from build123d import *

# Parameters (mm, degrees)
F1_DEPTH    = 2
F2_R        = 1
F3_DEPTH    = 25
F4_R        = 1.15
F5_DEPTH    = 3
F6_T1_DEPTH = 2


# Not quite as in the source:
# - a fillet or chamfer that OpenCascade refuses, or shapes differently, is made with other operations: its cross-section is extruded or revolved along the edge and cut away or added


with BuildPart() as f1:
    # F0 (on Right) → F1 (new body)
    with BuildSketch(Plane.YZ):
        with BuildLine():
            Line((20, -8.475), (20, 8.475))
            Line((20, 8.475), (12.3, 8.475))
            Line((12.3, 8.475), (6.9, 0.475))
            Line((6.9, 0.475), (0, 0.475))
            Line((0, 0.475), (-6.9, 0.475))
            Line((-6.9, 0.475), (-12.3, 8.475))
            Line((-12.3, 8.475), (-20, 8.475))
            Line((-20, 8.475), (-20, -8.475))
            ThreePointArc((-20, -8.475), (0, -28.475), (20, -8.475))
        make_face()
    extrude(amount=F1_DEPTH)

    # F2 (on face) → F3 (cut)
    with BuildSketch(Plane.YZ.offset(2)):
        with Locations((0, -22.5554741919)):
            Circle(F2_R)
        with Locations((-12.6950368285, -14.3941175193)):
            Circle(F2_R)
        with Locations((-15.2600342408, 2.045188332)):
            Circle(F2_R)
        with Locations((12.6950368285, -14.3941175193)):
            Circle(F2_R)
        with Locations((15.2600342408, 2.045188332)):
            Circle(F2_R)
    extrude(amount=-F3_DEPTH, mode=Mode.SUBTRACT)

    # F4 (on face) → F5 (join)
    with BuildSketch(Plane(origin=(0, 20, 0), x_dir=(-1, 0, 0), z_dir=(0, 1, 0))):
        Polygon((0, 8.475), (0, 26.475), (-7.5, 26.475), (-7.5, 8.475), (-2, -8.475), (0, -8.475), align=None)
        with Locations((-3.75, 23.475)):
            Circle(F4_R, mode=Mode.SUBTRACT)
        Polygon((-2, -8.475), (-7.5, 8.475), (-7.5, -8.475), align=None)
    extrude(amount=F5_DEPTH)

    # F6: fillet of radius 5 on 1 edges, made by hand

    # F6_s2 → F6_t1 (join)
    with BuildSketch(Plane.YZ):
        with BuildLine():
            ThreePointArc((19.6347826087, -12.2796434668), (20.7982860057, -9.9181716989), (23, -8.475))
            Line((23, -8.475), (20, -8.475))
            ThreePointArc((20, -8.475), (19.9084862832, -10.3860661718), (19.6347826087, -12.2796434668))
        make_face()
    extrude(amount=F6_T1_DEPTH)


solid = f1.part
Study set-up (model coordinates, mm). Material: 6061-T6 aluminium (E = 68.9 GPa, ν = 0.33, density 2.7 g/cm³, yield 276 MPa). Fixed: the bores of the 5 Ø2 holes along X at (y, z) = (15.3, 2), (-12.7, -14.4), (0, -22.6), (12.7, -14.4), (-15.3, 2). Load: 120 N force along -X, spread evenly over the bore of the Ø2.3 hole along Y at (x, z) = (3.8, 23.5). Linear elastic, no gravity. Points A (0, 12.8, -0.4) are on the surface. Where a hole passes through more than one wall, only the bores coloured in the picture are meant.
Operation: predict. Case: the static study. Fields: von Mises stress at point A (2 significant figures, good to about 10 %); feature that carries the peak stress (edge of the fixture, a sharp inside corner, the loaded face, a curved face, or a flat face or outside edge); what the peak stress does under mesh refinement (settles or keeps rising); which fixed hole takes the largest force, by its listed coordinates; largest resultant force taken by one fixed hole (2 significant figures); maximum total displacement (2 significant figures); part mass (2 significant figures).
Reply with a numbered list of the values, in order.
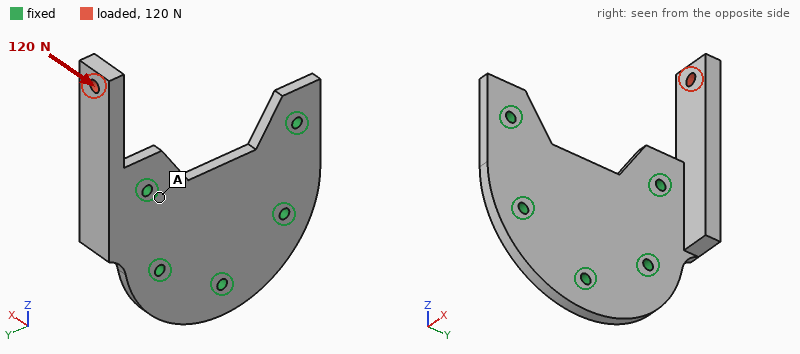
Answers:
1. 24 MPa
2. edge of the fixture
3. keeps rising
4. (15.3, 2)
5. 250 N
6. 0.25 mm
7. 8.2 g
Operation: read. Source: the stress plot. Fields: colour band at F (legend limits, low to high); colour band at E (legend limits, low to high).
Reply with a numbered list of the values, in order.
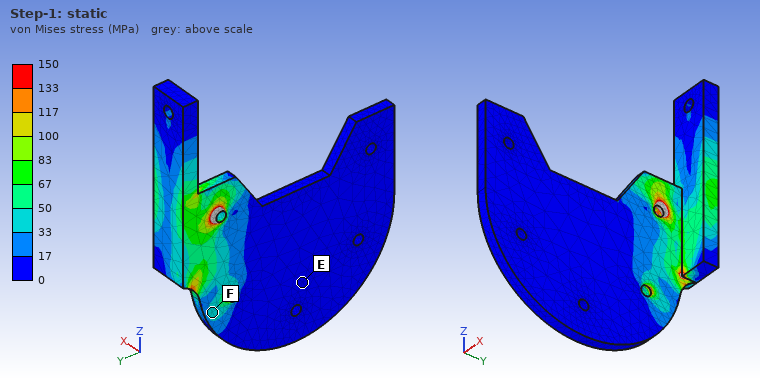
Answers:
1. 33 to 50 MPa
2. 0 to 17 MPa
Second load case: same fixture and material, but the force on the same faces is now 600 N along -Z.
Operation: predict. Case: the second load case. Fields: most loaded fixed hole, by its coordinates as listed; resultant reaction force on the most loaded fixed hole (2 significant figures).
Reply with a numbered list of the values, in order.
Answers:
1. (15.3, 2)
2. 480 N
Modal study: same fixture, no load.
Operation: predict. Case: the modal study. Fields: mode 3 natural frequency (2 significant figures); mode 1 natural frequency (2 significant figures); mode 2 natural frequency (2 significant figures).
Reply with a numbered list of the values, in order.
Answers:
1. 9600 Hz
2. 4400 Hz
3. 5600 Hz
